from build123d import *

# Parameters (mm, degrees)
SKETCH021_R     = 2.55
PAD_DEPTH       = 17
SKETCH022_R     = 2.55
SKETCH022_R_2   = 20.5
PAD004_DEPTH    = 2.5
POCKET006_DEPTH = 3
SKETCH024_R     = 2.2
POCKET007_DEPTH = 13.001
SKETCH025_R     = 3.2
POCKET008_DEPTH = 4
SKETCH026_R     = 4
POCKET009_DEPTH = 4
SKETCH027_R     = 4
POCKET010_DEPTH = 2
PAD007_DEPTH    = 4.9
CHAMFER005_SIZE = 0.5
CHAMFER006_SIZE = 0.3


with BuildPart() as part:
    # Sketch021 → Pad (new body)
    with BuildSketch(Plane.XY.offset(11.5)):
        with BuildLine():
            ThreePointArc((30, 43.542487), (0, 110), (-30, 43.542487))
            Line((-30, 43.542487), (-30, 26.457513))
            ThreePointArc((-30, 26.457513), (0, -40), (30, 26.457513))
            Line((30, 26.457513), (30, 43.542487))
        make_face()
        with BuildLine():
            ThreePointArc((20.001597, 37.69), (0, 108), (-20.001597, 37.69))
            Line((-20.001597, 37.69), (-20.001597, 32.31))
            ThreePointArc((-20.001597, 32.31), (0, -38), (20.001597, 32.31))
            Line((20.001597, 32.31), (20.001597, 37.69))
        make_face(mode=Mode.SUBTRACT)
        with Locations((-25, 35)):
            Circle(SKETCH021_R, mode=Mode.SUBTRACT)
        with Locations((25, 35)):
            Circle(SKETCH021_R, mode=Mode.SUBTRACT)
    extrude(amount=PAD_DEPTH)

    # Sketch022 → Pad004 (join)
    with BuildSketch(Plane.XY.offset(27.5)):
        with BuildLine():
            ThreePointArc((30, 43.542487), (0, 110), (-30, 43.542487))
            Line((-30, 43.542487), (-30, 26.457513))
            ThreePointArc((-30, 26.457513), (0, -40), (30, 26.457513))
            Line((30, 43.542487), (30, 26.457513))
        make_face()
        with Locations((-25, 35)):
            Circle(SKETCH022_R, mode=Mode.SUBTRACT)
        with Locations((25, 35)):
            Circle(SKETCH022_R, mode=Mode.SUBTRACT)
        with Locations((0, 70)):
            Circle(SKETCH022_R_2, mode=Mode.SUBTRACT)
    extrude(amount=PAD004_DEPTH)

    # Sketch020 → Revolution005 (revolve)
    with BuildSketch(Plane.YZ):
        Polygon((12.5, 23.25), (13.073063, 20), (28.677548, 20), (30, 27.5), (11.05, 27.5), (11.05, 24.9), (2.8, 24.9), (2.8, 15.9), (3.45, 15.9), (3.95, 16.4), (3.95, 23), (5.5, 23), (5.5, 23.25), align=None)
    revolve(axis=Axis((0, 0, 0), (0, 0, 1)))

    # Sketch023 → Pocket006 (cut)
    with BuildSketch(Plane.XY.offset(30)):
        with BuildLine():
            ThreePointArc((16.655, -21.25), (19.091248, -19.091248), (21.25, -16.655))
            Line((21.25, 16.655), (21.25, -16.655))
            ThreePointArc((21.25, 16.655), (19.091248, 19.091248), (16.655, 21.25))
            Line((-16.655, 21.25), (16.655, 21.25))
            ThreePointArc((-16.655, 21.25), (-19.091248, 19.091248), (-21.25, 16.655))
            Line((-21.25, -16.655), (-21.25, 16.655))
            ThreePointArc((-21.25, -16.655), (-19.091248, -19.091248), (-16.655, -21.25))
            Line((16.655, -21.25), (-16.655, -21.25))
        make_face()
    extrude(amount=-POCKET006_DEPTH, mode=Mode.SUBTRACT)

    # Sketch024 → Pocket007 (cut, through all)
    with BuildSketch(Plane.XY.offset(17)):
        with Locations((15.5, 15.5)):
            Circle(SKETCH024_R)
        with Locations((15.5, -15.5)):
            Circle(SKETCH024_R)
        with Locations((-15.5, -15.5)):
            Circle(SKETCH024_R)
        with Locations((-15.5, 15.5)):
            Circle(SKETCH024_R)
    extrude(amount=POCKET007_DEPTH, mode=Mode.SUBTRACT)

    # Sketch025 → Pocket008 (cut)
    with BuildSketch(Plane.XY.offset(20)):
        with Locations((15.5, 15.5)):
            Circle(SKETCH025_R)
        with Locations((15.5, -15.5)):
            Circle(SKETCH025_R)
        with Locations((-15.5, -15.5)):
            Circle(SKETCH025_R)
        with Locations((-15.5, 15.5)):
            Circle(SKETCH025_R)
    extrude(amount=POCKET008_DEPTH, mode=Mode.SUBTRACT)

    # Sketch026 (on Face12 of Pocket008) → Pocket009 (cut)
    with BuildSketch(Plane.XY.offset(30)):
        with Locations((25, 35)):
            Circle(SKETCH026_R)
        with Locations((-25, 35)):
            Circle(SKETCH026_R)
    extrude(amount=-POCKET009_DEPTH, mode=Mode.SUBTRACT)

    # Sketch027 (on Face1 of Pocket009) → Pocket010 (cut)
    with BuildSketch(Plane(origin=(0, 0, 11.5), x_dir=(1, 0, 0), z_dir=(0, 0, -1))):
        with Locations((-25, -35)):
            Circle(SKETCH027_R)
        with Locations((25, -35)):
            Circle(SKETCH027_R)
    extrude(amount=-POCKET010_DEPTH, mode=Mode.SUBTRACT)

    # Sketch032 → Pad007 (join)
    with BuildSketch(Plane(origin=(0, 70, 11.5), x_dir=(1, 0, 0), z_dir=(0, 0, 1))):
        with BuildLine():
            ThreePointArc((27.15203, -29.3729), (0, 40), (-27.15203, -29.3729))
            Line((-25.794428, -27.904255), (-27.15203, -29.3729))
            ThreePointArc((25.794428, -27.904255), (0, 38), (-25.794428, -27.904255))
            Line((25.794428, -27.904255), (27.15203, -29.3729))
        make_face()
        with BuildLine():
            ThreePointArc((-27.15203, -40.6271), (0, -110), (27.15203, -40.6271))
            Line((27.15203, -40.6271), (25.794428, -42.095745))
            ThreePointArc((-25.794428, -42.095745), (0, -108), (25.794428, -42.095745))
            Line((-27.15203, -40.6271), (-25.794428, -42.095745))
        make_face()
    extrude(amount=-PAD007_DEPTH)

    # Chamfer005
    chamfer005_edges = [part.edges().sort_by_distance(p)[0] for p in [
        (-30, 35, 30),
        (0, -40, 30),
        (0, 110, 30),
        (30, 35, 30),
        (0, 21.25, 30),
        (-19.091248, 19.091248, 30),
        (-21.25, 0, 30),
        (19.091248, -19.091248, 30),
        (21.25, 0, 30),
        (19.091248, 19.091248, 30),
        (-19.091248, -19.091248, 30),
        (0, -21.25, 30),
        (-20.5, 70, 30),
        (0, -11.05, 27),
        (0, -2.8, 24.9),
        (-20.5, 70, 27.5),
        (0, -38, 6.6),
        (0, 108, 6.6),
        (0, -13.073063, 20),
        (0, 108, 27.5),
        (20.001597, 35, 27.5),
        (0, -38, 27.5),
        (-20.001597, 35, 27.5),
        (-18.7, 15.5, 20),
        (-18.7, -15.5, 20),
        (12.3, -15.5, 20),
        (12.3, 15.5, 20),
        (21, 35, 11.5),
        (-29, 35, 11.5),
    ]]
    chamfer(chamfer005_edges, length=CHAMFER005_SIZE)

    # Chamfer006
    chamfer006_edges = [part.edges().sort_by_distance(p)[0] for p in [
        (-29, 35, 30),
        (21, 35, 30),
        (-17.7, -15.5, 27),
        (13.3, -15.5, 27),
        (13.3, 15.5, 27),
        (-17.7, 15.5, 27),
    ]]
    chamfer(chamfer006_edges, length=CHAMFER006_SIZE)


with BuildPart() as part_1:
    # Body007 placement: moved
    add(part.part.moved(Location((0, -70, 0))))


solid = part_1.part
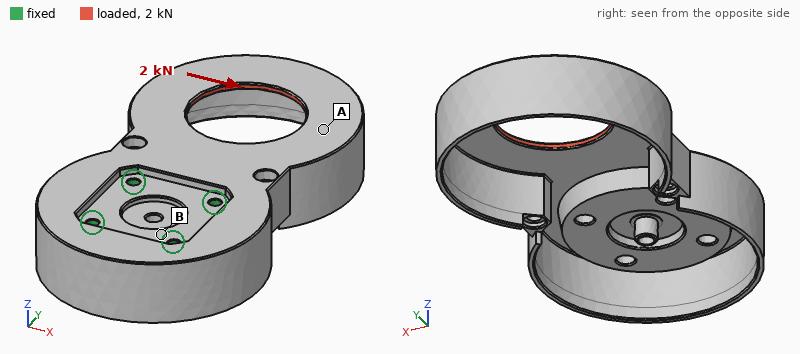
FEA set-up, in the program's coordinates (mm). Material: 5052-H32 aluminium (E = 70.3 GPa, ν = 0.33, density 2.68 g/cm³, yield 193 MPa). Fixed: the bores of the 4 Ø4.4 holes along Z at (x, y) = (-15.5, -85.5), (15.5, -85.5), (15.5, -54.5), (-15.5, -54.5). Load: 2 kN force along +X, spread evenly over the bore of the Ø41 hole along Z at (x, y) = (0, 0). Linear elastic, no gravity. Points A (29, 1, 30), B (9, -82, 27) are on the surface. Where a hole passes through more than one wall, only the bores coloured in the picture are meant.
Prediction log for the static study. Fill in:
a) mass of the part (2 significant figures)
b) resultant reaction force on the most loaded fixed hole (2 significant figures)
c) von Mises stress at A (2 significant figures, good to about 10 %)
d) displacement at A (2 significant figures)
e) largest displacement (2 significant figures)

140 g
2.3 kN
20 MPa
0.13 mm
0.26 mm
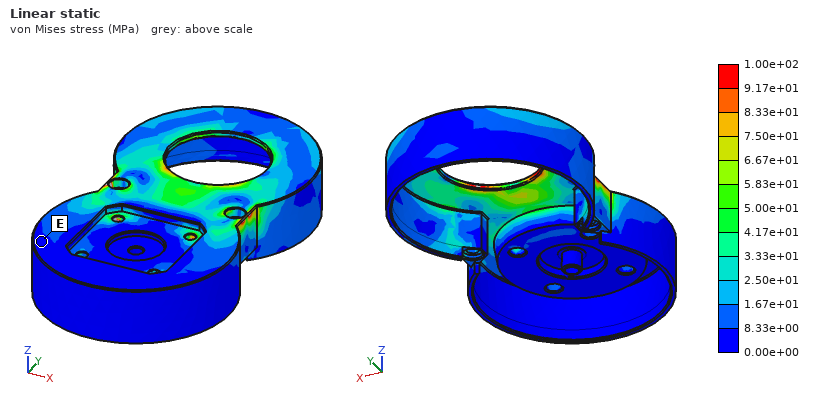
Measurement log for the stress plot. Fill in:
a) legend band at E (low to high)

0.00e+00 to 8.33e+00 MPa
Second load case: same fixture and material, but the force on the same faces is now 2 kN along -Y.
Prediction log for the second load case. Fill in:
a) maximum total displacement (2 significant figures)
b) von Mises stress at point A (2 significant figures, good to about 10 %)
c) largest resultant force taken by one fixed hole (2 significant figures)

0.10 mm
9.6 MPa
830 N
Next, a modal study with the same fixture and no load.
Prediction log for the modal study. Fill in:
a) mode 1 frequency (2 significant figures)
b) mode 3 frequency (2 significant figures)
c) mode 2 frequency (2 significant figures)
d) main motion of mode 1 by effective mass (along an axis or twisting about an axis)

470 Hz
1900 Hz
790 Hz
along Z
